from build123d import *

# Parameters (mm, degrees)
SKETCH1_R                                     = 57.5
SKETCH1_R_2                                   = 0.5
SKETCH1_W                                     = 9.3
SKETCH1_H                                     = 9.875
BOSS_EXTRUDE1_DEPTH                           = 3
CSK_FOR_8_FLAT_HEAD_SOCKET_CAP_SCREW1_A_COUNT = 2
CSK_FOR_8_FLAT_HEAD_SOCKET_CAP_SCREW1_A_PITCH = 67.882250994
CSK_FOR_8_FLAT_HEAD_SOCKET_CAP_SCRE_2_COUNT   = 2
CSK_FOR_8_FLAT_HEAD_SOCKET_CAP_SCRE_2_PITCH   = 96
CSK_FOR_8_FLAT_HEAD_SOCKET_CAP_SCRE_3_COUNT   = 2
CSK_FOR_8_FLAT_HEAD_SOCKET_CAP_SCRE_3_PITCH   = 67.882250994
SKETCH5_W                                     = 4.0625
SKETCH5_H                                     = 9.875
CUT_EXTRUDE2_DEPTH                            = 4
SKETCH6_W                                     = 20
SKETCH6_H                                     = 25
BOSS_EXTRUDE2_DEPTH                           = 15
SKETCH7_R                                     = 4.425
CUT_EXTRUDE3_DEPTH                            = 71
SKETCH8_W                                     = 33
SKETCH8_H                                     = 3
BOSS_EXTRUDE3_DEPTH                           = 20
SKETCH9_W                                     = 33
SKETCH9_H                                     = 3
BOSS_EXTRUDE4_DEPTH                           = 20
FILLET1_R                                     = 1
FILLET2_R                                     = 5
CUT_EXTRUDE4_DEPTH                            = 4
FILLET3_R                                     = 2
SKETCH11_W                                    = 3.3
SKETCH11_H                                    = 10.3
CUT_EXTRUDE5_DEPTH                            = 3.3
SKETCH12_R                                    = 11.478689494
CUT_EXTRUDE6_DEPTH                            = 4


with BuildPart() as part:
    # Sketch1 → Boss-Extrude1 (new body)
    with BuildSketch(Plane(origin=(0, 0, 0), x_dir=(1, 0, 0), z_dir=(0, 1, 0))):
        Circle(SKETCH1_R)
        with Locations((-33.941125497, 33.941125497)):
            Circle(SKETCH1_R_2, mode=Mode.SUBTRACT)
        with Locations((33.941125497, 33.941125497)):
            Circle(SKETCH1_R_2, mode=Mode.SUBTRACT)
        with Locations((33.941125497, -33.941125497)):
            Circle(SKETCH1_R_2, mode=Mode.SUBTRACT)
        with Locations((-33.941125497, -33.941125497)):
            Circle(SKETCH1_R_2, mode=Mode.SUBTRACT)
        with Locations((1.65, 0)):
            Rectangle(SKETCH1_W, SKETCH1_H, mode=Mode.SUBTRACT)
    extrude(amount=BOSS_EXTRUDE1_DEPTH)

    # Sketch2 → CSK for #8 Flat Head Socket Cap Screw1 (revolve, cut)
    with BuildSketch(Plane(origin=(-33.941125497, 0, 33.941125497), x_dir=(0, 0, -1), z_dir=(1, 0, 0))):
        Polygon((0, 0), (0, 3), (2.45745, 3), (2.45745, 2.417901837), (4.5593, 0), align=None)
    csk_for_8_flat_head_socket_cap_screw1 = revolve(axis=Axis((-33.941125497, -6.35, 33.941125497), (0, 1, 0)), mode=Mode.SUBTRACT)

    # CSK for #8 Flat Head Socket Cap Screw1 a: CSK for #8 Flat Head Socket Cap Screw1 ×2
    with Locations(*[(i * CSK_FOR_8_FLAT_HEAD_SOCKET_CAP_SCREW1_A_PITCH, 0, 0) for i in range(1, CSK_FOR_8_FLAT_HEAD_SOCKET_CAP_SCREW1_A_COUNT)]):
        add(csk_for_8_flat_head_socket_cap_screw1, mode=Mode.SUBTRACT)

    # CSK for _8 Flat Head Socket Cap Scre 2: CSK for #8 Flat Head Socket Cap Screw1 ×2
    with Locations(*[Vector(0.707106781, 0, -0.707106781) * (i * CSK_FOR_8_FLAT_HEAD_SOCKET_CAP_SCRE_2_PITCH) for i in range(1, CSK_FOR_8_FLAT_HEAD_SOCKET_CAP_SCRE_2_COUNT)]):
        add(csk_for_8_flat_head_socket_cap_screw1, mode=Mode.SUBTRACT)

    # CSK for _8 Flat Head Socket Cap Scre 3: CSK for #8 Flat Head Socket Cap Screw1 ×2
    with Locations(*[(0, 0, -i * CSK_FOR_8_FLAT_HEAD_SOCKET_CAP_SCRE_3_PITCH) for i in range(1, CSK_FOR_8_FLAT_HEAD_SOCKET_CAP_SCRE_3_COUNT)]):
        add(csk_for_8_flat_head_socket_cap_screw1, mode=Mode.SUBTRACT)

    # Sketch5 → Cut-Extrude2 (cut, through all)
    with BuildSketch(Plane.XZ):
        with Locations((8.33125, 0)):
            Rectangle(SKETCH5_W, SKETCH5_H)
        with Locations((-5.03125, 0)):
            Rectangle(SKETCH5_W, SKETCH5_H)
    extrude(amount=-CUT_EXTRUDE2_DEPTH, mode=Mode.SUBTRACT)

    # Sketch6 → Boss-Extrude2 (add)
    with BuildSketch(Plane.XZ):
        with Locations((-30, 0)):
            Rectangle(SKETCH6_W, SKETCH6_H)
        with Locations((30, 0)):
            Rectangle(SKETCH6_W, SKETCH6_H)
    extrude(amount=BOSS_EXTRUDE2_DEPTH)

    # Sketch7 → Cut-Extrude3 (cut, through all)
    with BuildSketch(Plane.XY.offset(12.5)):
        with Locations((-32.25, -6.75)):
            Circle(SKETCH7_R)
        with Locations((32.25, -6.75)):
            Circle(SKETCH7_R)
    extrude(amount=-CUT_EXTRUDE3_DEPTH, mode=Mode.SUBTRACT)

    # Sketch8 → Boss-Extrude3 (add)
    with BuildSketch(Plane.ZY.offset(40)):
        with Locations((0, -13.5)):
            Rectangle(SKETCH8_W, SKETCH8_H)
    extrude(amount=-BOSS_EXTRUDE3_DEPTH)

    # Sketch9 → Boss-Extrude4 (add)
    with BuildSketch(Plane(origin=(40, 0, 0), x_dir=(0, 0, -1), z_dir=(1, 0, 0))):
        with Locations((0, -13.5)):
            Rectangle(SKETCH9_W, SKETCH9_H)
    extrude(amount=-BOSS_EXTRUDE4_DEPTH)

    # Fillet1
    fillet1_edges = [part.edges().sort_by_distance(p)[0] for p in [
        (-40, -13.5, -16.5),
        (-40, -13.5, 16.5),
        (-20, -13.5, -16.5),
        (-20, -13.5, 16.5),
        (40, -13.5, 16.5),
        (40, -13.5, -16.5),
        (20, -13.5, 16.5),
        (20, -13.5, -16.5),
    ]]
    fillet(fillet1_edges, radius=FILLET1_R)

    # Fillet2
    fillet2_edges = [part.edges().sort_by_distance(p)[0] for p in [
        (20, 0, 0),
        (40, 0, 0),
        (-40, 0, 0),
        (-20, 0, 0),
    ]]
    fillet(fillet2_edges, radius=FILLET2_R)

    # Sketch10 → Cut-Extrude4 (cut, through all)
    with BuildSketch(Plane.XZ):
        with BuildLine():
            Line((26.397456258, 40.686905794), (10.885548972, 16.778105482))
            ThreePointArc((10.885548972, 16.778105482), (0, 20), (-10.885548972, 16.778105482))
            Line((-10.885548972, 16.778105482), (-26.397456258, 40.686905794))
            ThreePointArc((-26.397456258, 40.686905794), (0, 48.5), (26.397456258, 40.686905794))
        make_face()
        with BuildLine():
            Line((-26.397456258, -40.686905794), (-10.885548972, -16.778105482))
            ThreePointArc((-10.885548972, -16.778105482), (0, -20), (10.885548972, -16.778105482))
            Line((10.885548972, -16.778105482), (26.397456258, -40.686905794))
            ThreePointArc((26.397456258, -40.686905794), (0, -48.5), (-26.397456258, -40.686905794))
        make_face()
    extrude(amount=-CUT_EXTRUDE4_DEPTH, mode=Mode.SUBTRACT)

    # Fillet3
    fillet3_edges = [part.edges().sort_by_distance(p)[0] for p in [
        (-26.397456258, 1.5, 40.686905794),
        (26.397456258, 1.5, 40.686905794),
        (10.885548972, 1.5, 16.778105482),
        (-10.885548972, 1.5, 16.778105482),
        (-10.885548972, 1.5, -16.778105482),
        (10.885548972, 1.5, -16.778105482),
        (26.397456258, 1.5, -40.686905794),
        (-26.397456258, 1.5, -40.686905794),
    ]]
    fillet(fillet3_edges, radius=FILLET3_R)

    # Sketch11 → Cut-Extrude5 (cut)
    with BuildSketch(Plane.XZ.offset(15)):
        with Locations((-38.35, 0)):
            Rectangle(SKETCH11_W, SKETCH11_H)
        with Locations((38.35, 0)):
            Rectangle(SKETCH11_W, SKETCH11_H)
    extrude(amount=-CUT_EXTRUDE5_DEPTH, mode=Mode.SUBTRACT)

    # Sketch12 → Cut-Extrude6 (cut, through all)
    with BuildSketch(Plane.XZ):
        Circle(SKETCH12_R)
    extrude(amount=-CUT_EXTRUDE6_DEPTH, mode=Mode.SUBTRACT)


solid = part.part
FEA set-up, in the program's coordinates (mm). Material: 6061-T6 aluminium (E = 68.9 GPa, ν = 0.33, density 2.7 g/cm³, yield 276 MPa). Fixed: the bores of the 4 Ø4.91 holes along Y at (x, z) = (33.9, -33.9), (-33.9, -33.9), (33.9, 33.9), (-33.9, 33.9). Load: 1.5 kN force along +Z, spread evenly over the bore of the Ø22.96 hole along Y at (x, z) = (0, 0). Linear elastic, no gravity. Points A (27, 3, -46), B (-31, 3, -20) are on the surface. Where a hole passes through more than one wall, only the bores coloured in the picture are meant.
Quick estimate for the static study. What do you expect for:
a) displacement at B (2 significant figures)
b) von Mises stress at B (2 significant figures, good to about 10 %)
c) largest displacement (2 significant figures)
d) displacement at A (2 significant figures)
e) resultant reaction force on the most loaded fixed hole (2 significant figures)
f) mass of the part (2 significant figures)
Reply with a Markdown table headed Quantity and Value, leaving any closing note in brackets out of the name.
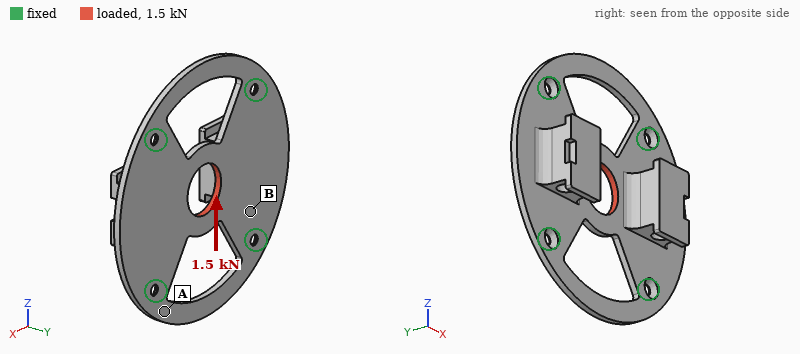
| Quantity | Value |
|---|---|
| displacement at B | 4.6 µm |
| von Mises stress at B | 8.9 MPa |
| largest displacement | 13 µm |
| displacement at A | 5.3 µm |
| resultant reaction force on the most loaded fixed hole | 420 N |
| mass of the part | 97 g |
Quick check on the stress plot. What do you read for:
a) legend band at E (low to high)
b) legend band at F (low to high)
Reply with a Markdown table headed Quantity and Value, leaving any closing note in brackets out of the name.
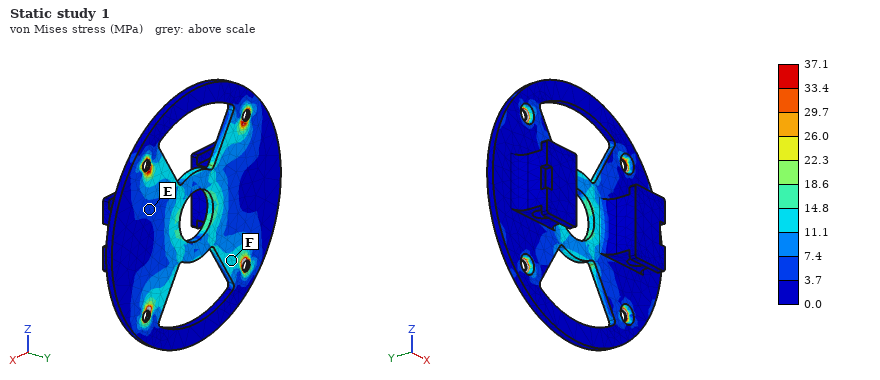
| Quantity | Value |
|---|---|
| legend band at E | 3.7 to 7.4 MPa |
| legend band at F | 11.1 to 14.8 MPa |
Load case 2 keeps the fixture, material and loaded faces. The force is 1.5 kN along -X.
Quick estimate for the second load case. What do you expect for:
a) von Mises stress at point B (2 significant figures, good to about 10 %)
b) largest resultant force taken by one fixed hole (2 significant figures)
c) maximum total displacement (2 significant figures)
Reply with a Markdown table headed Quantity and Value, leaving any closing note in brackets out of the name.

| Quantity | Value |
|---|---|
| von Mises stress at point B | 8.3 MPa |
| largest resultant force taken by one fixed hole | 380 N |
| maximum total displacement | 11 µm |
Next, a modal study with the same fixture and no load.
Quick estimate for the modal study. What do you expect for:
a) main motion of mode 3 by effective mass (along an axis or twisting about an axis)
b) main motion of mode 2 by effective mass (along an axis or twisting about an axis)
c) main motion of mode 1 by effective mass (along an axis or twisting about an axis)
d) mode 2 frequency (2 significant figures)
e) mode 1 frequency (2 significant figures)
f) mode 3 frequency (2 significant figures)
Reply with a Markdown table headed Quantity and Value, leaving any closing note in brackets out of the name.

| Quantity | Value |
|---|---|
| main motion of mode 3 by effective mass | twisting about X |
| main motion of mode 2 by effective mass | along Y |
| main motion of mode 1 by effective mass | along Y |
| mode 2 frequency | 2000 Hz |
| mode 1 frequency | 1500 Hz |
| mode 3 frequency | 2100 Hz |
